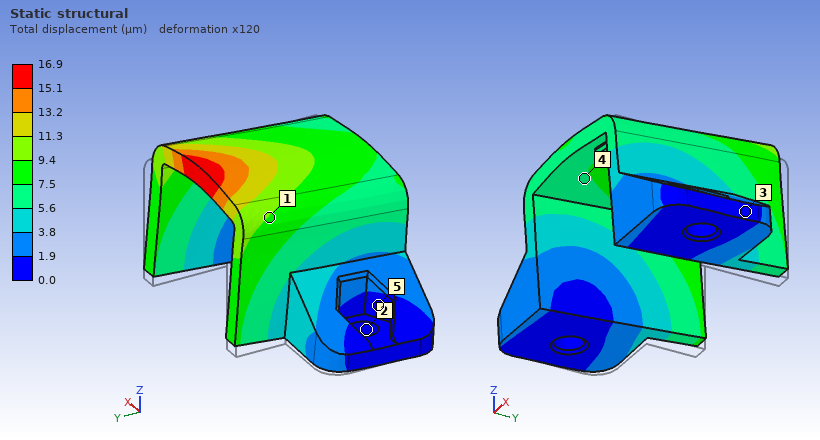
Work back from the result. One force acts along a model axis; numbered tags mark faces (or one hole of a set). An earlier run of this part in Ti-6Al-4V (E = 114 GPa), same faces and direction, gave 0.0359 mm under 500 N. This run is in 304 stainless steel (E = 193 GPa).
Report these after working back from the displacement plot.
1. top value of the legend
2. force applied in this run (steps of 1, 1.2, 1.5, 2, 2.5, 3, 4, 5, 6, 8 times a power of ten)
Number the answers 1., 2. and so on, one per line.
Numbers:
1. 16.9 µm
2. 400 N
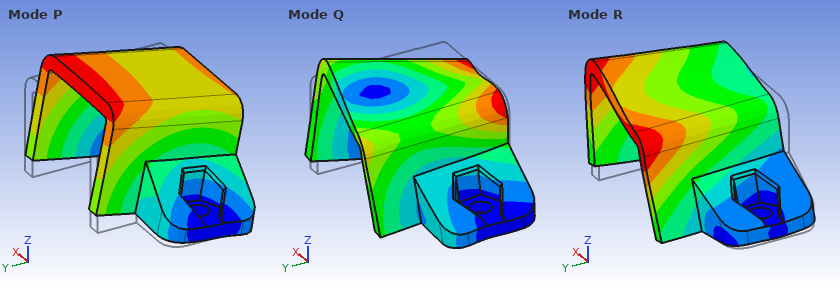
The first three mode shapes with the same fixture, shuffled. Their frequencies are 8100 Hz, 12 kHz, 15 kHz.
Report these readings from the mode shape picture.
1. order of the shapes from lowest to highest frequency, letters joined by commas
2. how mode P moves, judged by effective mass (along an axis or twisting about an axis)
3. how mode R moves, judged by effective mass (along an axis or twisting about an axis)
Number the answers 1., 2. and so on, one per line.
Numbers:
1. P, R, Q
2. along Y
3. along X
